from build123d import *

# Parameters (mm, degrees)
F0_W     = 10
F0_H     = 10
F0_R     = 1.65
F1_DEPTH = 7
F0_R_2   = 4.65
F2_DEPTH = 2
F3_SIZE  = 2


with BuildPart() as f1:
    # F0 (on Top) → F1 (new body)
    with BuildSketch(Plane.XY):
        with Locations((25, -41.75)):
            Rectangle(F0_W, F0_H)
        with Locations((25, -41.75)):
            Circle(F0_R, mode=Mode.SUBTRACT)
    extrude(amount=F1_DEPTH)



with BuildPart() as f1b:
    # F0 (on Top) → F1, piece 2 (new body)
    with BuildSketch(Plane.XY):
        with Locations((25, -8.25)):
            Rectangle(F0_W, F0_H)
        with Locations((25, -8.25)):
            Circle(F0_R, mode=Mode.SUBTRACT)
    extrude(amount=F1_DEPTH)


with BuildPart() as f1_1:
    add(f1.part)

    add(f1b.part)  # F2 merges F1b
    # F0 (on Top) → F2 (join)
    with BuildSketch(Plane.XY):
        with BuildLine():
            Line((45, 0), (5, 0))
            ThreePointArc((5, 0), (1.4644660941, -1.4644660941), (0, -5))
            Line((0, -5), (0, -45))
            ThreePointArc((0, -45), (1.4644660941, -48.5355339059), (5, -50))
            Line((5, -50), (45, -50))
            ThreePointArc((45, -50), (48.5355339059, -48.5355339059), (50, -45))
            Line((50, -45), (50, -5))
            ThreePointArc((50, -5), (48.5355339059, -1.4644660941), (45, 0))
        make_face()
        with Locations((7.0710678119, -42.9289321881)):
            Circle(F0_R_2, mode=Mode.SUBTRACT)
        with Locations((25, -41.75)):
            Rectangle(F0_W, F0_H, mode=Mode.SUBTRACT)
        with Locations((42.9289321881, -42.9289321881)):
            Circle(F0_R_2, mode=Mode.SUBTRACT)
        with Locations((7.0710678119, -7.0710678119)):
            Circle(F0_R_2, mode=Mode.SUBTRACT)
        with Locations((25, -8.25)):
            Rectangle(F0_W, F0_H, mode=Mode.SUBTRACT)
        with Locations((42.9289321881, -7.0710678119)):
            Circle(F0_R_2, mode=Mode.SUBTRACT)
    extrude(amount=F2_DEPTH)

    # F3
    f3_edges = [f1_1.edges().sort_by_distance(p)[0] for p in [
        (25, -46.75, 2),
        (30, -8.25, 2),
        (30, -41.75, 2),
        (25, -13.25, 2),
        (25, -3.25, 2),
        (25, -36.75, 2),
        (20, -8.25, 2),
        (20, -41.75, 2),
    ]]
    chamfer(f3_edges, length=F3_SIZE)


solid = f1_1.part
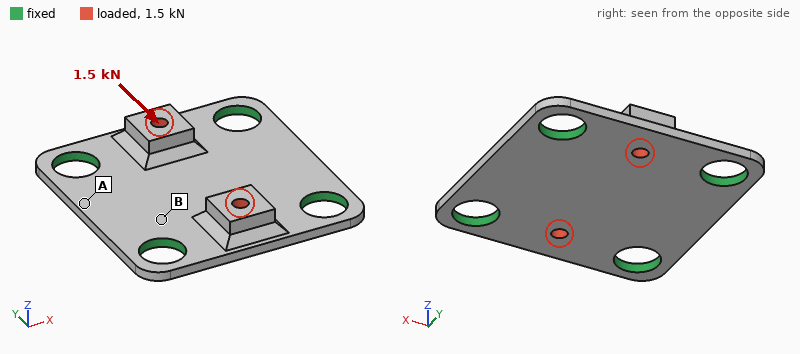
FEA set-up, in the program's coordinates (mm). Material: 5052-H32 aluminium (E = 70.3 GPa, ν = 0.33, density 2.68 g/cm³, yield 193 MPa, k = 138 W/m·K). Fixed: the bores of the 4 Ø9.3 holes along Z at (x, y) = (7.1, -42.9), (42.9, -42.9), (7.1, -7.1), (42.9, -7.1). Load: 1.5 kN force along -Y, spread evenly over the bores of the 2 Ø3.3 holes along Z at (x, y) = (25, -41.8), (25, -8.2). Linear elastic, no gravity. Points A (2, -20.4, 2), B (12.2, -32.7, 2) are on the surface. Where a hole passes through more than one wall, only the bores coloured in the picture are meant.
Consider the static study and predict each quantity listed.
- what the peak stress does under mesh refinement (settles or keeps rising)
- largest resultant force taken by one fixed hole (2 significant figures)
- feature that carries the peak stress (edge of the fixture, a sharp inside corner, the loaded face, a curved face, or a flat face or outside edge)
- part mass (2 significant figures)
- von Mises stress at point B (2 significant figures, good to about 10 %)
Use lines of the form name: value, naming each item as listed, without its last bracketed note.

what the peak stress does under mesh refinement: keeps rising
largest resultant force taken by one fixed hole: 400 N
feature that carries the peak stress: edge of the fixture
part mass: 15 g
von Mises stress at point B: 10 MPa
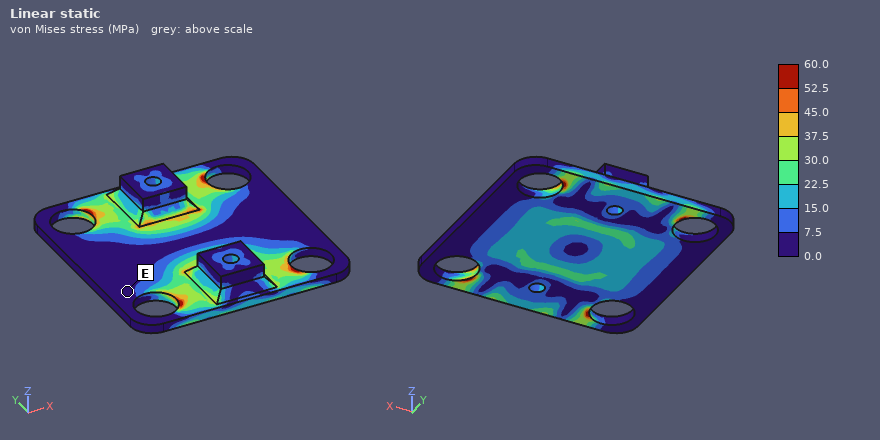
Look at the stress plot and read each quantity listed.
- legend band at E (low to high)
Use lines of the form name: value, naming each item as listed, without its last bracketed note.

legend band at E: 0.0 to 7.5 MPa
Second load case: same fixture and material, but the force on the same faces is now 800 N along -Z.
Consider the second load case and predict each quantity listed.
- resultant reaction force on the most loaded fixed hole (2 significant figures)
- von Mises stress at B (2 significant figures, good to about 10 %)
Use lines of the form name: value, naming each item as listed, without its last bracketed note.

resultant reaction force on the most loaded fixed hole: 250 N
von Mises stress at B: 9.6 MPa
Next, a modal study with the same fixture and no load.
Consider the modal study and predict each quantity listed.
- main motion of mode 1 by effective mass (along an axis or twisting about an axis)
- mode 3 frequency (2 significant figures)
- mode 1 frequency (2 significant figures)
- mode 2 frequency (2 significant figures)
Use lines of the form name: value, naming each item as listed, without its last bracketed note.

main motion of mode 1 by effective mass: along Z
mode 3 frequency: 14 kHz
mode 1 frequency: 9100 Hz
mode 2 frequency: 14 kHz
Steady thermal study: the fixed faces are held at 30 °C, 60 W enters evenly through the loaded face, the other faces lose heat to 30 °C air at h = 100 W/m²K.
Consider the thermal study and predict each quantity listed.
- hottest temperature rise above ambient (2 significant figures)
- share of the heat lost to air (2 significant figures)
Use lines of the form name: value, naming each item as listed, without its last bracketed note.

hottest temperature rise above ambient: 36 K
share of the heat lost to air: 11 %
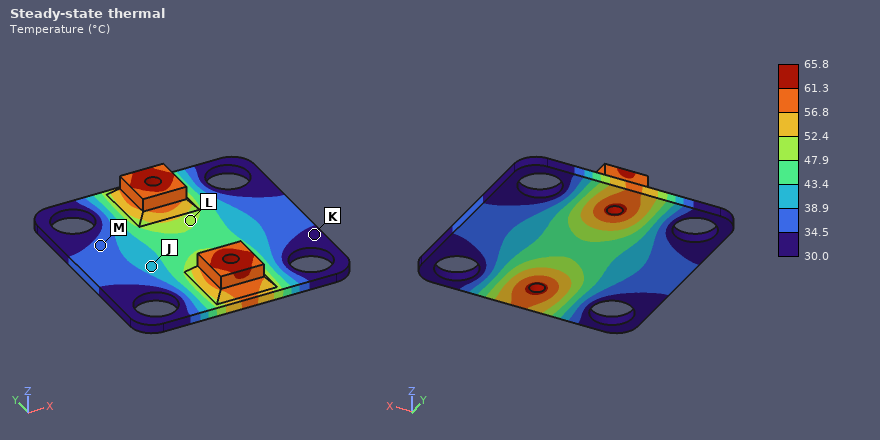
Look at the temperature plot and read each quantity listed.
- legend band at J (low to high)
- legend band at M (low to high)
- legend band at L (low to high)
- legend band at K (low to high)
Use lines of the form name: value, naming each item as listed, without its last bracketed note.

legend band at J: 38.9 to 43.4 °C
legend band at M: 34.5 to 38.9 °C
legend band at L: 47.9 to 52.4 °C
legend band at K: 30.0 to 34.5 °C
